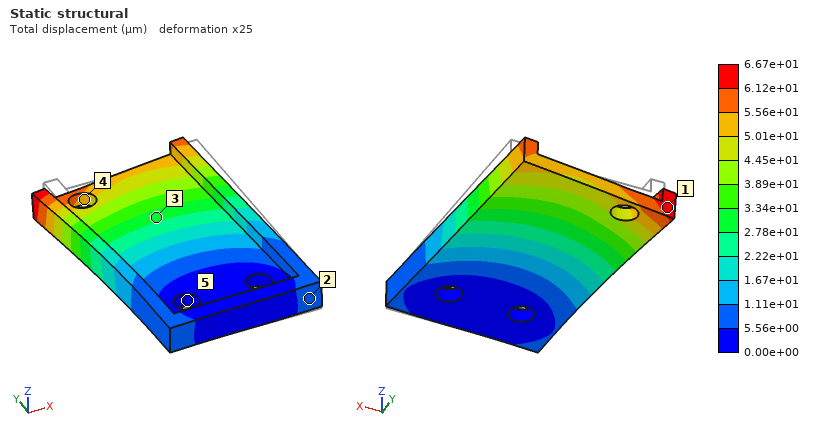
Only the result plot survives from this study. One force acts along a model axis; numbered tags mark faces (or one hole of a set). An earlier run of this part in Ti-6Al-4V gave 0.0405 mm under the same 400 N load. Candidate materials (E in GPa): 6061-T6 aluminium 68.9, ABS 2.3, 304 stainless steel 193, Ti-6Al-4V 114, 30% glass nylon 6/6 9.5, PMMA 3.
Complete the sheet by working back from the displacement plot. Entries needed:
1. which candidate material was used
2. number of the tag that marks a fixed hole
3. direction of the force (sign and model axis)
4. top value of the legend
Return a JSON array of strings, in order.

["6061-T6 aluminium", "5", "-X", "6.67e+01 µm"]
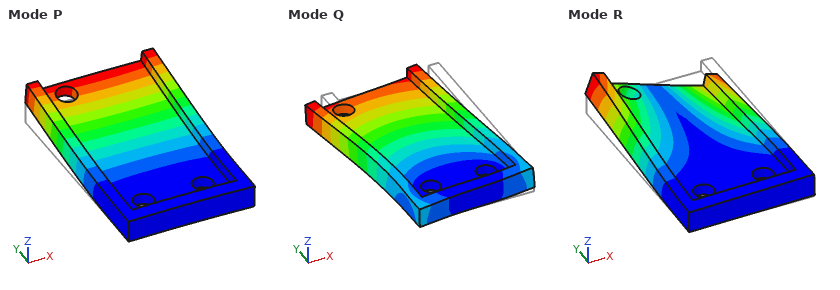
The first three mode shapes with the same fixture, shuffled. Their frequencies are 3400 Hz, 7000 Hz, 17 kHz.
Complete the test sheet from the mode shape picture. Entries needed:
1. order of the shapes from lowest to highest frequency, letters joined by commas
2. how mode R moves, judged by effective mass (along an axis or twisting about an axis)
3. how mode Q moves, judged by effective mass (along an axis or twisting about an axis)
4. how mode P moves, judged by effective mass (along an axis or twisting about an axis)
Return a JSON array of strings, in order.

["P, R, Q", "twisting about Y", "along X", "along Z"]
